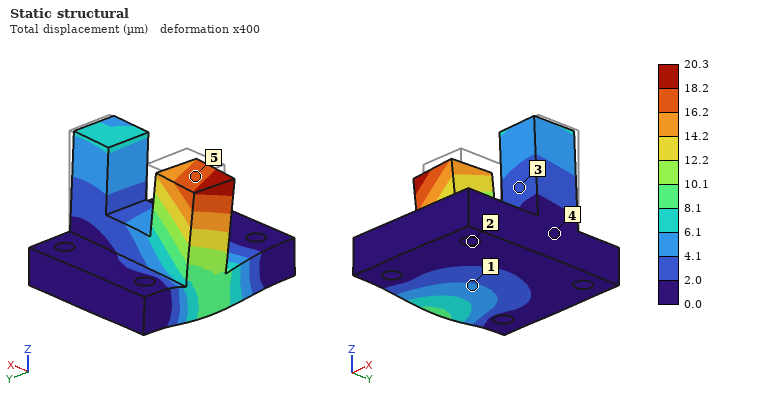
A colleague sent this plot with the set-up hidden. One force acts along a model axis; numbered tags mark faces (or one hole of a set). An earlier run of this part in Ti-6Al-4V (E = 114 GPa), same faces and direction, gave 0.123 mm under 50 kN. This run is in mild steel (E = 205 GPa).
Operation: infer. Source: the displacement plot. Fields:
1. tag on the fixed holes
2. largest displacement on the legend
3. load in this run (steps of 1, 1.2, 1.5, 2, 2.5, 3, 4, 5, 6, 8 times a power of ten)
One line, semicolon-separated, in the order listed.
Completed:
2; 20.3 µm; 15 kN
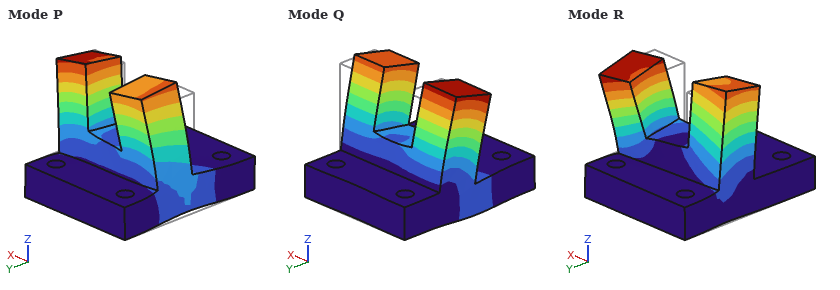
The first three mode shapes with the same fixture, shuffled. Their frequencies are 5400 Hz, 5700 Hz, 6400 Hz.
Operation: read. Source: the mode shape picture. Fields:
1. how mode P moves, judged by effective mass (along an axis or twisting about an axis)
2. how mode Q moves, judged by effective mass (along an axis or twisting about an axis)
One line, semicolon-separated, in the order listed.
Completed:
along X; along Y
